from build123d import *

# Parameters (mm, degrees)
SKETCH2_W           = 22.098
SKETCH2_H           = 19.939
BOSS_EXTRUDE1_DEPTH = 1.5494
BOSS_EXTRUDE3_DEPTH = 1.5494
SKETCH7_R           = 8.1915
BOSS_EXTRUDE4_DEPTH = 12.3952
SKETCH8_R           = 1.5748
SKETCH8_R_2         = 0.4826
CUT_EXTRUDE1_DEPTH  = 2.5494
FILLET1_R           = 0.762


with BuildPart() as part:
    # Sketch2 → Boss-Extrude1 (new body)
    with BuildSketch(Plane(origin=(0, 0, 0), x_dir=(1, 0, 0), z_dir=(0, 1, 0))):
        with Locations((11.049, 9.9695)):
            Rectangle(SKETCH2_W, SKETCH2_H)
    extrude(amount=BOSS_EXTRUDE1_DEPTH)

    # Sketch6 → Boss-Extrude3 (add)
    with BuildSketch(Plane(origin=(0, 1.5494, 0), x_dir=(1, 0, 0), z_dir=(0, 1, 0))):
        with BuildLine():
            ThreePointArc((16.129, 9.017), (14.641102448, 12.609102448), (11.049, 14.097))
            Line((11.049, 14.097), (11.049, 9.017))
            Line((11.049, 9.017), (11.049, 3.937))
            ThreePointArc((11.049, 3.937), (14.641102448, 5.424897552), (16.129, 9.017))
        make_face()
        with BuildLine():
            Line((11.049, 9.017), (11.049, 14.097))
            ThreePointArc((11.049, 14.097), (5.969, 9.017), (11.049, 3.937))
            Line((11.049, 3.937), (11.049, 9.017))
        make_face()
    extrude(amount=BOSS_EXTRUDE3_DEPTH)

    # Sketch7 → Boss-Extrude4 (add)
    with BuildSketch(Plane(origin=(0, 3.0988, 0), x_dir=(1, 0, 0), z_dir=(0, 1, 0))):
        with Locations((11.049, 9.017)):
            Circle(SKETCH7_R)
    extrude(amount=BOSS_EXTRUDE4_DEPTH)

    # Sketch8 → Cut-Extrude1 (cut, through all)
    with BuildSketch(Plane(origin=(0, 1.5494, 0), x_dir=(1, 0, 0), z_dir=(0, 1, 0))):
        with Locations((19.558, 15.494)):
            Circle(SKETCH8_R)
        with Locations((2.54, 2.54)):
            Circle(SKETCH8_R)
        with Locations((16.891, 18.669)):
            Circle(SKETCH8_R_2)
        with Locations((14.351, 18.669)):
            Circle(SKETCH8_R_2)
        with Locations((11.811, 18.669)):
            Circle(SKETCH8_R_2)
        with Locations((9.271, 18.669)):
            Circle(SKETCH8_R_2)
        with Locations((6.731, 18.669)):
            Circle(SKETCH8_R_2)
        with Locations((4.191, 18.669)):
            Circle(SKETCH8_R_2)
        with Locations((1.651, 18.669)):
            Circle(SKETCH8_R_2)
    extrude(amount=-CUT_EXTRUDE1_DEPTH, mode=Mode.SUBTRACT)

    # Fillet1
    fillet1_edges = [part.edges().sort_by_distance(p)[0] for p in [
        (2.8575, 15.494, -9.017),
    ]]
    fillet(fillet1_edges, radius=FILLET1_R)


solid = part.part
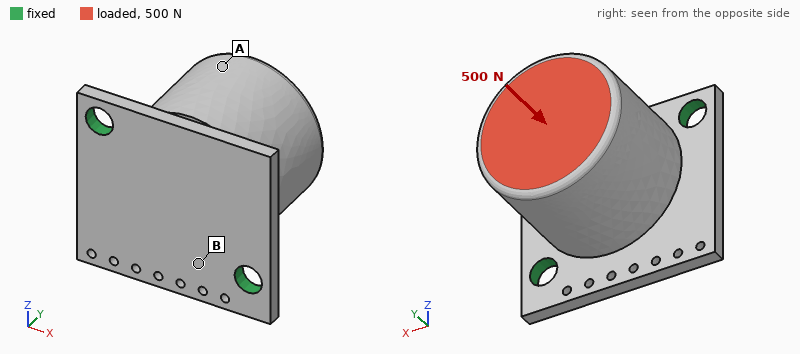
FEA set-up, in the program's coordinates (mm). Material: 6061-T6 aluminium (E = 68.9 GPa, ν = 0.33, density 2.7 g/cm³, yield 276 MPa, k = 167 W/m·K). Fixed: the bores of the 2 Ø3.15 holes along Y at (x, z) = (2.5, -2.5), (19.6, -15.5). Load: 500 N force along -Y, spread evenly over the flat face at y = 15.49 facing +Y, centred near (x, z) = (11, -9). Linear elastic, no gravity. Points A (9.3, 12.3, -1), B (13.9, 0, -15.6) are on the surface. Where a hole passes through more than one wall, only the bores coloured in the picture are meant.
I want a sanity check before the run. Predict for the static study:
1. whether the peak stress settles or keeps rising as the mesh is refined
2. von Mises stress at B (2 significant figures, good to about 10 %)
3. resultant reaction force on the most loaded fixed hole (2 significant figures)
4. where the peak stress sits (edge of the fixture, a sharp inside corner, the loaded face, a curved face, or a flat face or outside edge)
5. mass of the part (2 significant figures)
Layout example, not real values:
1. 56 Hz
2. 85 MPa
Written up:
1. keeps rising
2. 40 MPa
3. 270 N
4. edge of the fixture
5. 9.1 g
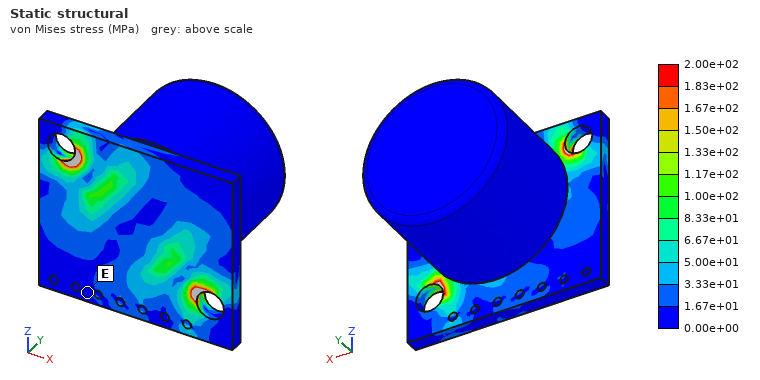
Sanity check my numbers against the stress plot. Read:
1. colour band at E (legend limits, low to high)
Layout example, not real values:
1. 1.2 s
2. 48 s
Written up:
1. 0.00e+00 to 1.67e+01 MPa
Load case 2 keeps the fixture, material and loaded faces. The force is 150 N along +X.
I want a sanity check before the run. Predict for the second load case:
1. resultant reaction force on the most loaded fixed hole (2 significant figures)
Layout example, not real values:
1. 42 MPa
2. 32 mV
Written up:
1. 140 N
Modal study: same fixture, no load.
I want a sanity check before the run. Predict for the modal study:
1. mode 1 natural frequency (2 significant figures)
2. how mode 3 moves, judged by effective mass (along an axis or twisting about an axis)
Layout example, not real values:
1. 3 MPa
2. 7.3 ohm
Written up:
1. 2400 Hz
2. along Y
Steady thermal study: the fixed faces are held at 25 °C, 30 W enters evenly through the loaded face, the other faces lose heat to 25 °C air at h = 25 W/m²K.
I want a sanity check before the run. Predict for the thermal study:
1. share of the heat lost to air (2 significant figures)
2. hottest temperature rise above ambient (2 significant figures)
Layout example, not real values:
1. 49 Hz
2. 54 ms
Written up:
1. 4.8 %
2. 51 K
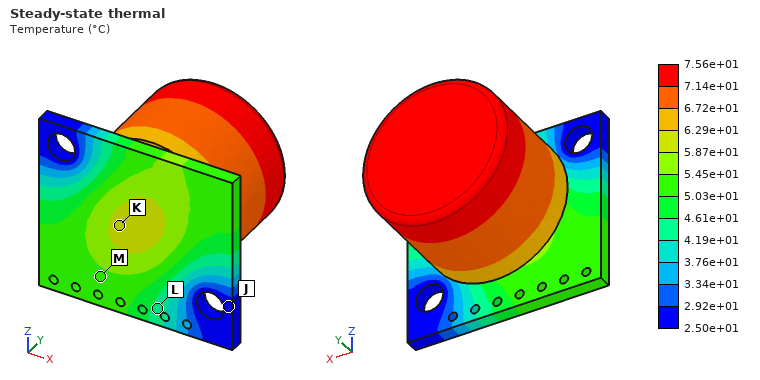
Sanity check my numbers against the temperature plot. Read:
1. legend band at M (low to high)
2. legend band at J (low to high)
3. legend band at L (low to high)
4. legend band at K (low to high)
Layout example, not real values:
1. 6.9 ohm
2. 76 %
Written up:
1. 5.03e+01 to 5.45e+01 °C
2. 2.50e+01 to 2.92e+01 °C
3. 4.19e+01 to 4.61e+01 °C
4. 5.87e+01 to 6.29e+01 °C
